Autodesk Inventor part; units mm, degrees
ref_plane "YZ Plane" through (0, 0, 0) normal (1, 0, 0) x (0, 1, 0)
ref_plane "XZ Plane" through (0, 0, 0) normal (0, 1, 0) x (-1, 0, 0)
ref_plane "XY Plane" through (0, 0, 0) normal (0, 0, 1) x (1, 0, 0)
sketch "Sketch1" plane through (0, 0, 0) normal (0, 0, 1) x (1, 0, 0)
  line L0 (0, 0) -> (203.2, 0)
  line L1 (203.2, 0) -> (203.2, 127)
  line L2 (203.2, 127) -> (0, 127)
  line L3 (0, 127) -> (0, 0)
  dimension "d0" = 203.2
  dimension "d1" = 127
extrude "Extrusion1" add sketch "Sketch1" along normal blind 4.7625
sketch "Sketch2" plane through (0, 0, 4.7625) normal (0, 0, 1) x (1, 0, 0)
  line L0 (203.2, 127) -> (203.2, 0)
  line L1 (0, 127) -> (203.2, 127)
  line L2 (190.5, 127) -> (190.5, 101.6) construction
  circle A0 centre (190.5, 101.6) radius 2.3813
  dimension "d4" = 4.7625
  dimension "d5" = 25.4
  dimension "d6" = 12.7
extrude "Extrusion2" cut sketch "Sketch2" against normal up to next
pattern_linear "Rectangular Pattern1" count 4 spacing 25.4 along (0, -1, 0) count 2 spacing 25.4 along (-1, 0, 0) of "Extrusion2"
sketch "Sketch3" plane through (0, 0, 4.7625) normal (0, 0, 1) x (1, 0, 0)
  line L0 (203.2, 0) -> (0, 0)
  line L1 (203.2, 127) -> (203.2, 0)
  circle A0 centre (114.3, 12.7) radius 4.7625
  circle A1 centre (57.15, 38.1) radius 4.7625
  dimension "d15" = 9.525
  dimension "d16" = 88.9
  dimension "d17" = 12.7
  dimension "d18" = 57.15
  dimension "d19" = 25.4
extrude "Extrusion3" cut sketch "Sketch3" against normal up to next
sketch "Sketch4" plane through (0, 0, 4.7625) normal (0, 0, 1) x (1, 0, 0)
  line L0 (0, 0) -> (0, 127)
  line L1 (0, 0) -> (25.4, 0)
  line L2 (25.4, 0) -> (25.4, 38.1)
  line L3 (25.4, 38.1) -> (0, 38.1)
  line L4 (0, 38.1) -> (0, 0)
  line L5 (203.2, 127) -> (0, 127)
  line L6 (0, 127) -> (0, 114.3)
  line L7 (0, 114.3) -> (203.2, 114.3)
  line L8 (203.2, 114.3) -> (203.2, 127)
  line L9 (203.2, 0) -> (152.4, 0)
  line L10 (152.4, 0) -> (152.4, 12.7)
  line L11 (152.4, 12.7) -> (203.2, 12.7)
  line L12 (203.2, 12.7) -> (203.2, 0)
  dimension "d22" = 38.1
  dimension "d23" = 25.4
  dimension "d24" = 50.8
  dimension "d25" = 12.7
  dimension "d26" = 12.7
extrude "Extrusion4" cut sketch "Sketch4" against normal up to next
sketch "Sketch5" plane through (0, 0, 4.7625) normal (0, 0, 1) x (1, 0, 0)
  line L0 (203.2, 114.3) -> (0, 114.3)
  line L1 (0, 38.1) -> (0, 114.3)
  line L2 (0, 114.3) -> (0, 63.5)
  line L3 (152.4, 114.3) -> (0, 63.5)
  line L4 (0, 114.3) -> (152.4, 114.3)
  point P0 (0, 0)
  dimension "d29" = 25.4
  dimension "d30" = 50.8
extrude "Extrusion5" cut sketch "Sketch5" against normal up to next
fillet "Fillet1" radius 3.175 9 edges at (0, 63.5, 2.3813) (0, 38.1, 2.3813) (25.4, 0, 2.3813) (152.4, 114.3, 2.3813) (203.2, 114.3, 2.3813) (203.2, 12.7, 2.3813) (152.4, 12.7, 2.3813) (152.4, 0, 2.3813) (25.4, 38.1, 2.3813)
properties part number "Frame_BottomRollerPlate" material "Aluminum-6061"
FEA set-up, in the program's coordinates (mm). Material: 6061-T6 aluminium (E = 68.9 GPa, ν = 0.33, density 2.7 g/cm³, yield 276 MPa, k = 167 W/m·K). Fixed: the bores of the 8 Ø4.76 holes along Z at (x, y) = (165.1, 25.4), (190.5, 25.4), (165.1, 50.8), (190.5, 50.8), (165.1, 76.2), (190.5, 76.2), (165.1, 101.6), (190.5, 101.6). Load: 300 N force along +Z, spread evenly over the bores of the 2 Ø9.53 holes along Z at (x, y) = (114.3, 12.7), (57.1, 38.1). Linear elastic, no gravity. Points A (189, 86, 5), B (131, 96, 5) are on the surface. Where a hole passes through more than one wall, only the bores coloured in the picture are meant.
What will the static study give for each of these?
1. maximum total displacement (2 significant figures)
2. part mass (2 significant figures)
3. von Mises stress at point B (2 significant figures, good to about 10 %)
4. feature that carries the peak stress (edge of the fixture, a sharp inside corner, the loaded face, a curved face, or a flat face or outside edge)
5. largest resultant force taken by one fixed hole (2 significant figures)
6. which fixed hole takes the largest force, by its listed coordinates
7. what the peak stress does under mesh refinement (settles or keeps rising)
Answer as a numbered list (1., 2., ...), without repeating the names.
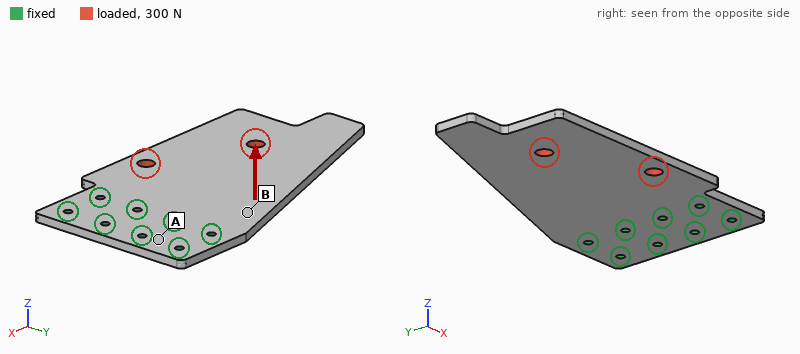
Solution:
1. 2.3 mm
2. 220 g
3. 36 MPa
4. edge of the fixture
5. 290 N
6. (165.1, 25.4)
7. keeps rising
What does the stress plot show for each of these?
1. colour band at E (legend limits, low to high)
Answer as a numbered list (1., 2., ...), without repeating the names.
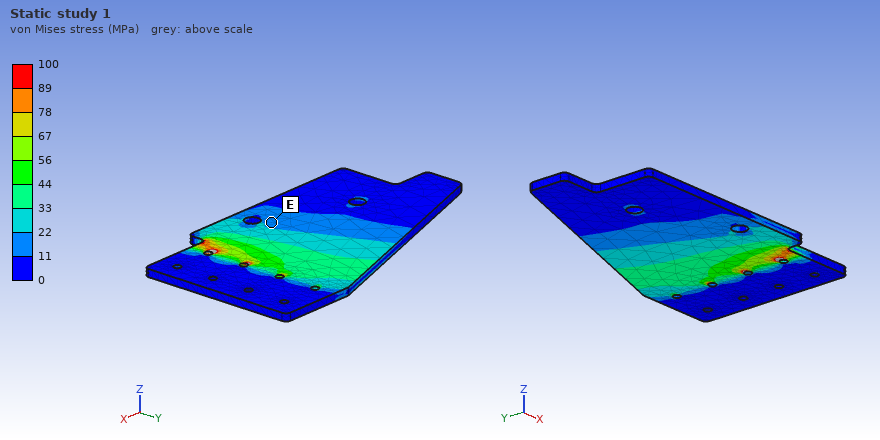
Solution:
1. 11 to 22 MPa
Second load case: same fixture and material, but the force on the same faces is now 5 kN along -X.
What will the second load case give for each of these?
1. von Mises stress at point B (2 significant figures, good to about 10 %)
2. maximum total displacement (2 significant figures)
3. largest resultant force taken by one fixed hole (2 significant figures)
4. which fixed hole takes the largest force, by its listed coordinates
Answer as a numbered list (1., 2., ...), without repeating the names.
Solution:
1. 4.9 MPa
2. 65 µm
3. 3.1 kN
4. (165.1, 25.4)
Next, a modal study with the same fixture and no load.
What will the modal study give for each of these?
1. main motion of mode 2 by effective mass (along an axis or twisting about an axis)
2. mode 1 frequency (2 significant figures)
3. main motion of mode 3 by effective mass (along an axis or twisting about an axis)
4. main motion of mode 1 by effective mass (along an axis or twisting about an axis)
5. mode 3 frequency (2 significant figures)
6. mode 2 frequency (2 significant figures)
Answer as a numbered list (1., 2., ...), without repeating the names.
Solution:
1. twisting about X
2. 190 Hz
3. along Z
4. along Z
5. 1000 Hz
6. 750 Hz
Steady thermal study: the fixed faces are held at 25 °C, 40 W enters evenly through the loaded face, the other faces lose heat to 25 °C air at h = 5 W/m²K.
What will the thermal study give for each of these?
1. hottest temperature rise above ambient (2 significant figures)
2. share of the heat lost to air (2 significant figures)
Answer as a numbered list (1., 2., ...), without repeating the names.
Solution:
1. 46 K
2. 9.7 %
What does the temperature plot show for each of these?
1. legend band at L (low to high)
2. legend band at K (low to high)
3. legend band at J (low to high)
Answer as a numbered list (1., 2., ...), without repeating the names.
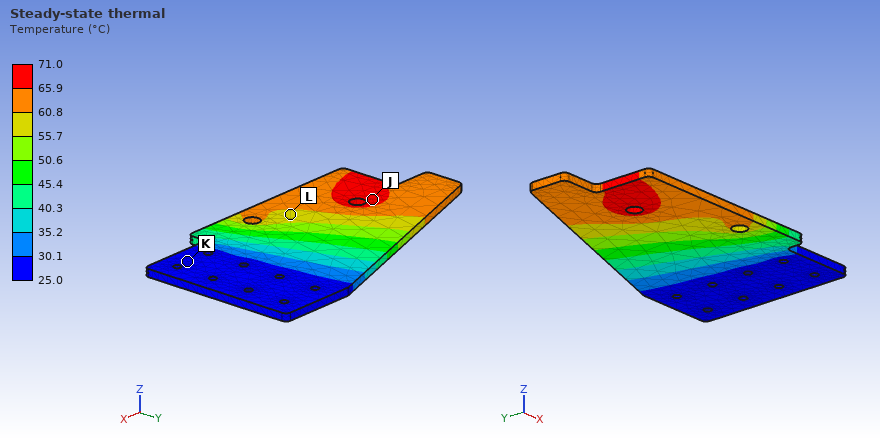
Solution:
1. 55.7 to 60.8 °C
2. 25.0 to 30.1 °C
3. 65.9 to 71.0 °C
